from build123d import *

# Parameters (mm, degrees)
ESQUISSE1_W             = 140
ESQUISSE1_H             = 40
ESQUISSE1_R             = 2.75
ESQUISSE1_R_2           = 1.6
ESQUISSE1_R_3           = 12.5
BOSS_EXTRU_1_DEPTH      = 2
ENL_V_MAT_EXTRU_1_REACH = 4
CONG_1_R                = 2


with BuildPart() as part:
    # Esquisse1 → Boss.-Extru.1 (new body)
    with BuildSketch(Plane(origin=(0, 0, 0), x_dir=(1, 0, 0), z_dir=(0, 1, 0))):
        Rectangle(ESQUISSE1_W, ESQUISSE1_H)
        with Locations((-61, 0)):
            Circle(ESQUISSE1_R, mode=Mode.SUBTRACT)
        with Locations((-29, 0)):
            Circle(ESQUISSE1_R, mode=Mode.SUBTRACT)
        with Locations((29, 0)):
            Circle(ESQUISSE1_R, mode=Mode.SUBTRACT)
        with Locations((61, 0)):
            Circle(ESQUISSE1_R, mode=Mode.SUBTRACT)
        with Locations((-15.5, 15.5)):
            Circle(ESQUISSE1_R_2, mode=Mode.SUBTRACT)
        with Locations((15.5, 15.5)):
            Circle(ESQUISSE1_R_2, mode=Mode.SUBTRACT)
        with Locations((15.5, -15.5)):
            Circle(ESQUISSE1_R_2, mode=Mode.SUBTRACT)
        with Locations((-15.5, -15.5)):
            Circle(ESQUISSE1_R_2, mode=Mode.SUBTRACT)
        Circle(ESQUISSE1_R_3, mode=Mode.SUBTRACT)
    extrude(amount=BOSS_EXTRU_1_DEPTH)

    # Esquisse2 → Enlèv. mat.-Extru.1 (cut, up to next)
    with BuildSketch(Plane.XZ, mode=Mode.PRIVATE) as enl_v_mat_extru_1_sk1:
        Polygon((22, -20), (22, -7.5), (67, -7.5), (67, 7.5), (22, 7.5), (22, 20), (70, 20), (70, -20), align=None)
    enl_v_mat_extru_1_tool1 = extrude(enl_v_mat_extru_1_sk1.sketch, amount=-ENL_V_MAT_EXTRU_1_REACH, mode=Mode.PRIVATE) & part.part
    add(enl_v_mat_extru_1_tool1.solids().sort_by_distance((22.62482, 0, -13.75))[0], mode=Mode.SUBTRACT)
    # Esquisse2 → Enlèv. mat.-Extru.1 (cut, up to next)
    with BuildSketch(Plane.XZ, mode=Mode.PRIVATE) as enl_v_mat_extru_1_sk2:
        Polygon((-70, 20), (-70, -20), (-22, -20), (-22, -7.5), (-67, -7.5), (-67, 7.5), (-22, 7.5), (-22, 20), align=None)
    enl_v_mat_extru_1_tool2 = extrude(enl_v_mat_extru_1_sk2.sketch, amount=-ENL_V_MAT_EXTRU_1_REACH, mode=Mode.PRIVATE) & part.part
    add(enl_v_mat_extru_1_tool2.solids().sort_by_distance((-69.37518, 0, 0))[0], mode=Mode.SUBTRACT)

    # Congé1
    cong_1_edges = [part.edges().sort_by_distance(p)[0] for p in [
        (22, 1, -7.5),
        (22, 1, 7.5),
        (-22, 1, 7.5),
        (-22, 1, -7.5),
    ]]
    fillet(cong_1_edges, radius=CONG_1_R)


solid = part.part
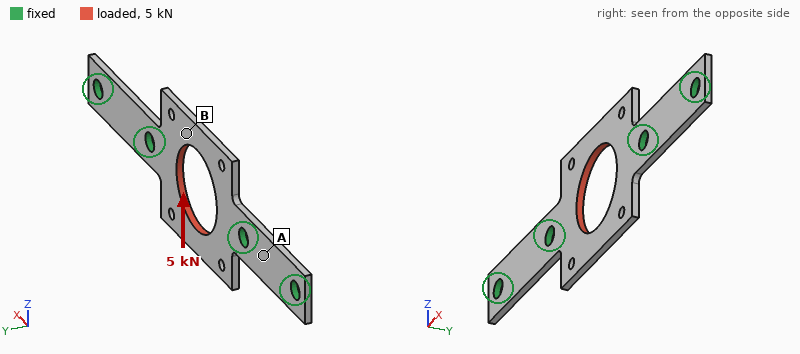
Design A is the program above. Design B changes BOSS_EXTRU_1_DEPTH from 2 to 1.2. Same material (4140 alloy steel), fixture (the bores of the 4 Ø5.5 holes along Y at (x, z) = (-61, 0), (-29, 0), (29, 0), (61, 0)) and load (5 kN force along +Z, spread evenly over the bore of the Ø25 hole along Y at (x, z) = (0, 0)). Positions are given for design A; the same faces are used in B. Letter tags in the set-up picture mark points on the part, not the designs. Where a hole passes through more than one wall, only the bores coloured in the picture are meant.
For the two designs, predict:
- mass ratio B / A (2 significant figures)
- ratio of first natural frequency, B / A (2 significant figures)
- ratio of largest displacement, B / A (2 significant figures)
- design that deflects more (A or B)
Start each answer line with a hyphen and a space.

- 0.60
- 0.62
- 1.7
- B
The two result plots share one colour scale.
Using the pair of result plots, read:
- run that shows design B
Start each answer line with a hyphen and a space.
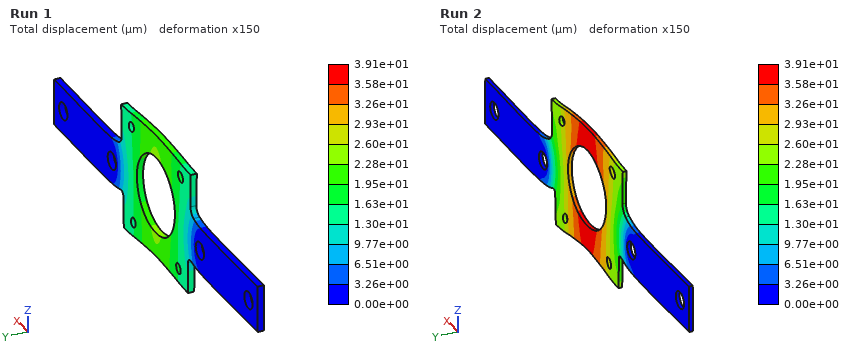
- Run 2
